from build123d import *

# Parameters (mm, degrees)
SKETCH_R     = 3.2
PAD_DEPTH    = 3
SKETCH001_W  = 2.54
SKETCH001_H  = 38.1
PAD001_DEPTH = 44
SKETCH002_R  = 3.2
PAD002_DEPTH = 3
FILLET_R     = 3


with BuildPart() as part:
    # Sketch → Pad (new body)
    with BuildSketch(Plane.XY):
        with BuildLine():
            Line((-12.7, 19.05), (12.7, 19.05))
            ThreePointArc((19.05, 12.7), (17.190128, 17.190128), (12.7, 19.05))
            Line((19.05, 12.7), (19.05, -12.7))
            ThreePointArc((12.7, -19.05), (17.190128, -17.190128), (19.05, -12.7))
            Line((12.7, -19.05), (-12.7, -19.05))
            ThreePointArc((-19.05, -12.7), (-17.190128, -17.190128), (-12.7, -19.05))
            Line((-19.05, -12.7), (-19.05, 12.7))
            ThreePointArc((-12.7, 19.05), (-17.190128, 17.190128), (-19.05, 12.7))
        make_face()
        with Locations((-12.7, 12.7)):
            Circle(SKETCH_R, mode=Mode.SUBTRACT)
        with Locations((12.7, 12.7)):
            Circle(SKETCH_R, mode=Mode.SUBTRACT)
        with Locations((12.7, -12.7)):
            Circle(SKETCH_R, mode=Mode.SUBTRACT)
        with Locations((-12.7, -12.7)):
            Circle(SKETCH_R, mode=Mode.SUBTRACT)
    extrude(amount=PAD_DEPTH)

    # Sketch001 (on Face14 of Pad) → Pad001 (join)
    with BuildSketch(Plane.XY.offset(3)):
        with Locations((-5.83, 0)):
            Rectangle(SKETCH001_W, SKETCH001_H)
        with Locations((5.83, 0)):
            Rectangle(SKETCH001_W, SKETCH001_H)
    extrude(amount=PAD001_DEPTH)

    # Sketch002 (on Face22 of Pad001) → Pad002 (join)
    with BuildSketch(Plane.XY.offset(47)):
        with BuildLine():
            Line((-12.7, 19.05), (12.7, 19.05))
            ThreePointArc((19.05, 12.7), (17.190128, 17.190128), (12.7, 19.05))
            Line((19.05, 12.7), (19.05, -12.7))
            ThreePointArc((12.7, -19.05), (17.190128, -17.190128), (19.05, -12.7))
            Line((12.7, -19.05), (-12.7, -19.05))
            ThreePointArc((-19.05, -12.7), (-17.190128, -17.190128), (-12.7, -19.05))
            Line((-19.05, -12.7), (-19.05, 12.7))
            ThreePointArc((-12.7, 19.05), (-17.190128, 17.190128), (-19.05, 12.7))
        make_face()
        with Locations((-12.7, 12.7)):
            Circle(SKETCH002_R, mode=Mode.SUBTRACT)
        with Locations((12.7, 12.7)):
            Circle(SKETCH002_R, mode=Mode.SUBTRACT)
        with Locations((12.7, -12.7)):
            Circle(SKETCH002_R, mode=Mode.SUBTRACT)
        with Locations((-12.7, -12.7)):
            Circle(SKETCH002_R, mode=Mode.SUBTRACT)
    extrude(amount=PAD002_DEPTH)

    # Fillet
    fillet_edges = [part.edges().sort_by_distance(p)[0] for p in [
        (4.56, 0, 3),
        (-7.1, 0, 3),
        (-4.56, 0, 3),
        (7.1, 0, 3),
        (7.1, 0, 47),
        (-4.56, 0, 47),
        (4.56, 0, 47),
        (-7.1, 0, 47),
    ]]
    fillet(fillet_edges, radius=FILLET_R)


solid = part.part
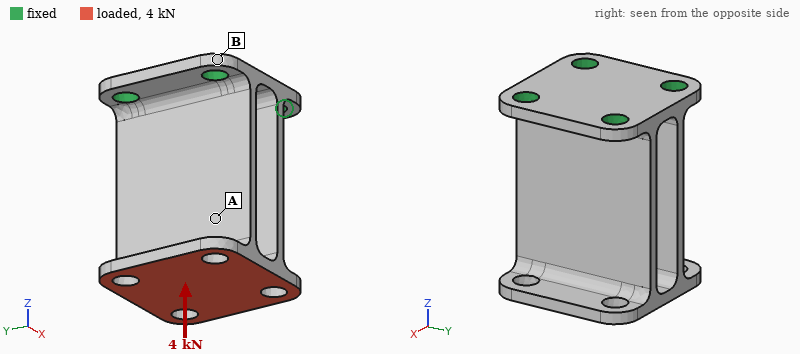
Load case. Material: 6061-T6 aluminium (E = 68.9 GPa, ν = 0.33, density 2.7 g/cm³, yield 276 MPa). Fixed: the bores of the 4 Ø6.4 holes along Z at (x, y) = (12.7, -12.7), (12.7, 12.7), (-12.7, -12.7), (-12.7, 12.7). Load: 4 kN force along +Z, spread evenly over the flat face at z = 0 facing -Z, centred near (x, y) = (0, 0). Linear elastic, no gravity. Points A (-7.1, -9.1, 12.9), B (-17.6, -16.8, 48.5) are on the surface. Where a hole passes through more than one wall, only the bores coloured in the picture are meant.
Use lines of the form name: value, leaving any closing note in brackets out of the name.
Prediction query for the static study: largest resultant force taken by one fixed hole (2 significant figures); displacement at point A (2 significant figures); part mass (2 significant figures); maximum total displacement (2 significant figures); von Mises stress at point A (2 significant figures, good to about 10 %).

largest resultant force taken by one fixed hole: 1.0 kN
displacement at point A: 0.040 mm
part mass: 45 g
maximum total displacement: 0.12 mm
von Mises stress at point A: 40 MPa
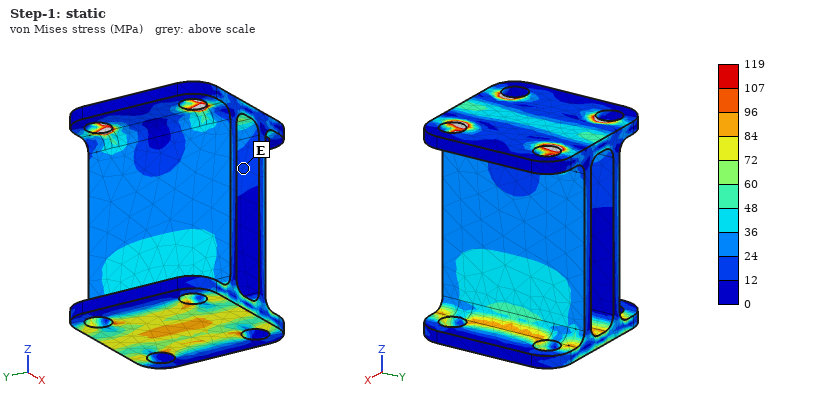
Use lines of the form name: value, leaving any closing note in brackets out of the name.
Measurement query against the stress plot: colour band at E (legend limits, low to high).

colour band at E: 12 to 24 MPa
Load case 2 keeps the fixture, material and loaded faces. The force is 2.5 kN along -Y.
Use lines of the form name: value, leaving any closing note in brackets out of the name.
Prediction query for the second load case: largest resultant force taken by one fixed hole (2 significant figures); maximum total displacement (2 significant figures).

largest resultant force taken by one fixed hole: 2.4 kN
maximum total displacement: 0.19 mm
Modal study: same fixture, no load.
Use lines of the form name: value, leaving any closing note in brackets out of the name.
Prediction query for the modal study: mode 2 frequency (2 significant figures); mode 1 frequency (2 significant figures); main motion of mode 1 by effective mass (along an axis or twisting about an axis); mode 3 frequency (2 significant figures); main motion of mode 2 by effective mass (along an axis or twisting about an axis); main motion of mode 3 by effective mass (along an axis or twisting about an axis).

mode 2 frequency: 3100 Hz
mode 1 frequency: 1200 Hz
main motion of mode 1 by effective mass: along X
mode 3 frequency: 4500 Hz
main motion of mode 2 by effective mass: twisting about Z
main motion of mode 3 by effective mass: along Y
